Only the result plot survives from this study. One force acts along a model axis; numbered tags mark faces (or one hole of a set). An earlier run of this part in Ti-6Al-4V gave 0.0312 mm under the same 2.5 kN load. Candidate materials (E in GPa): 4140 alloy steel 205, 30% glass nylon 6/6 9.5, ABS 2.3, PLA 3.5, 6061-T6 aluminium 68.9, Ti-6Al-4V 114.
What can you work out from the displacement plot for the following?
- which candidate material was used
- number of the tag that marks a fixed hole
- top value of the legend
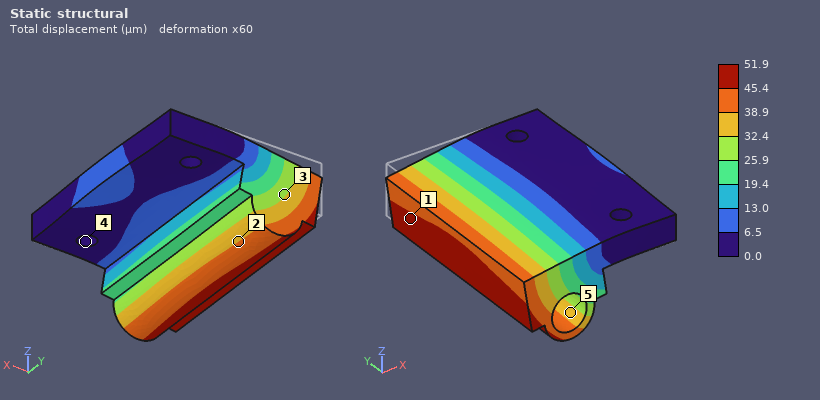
6061-T6 aluminium
4
51.9 µm
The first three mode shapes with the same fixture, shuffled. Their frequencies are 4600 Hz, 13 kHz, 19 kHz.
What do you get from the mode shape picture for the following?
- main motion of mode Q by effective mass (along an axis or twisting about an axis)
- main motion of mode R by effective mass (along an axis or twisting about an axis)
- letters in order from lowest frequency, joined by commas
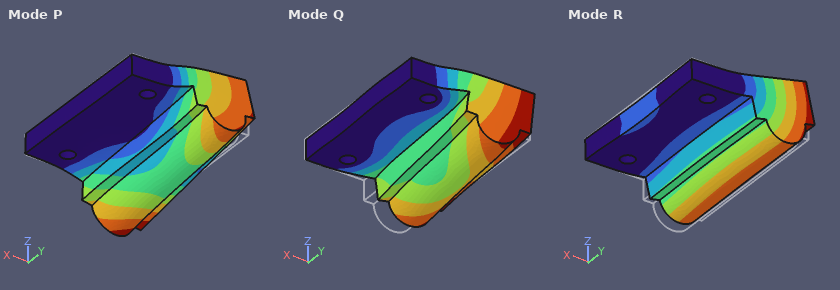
along Y
along Z
R, P, Q
